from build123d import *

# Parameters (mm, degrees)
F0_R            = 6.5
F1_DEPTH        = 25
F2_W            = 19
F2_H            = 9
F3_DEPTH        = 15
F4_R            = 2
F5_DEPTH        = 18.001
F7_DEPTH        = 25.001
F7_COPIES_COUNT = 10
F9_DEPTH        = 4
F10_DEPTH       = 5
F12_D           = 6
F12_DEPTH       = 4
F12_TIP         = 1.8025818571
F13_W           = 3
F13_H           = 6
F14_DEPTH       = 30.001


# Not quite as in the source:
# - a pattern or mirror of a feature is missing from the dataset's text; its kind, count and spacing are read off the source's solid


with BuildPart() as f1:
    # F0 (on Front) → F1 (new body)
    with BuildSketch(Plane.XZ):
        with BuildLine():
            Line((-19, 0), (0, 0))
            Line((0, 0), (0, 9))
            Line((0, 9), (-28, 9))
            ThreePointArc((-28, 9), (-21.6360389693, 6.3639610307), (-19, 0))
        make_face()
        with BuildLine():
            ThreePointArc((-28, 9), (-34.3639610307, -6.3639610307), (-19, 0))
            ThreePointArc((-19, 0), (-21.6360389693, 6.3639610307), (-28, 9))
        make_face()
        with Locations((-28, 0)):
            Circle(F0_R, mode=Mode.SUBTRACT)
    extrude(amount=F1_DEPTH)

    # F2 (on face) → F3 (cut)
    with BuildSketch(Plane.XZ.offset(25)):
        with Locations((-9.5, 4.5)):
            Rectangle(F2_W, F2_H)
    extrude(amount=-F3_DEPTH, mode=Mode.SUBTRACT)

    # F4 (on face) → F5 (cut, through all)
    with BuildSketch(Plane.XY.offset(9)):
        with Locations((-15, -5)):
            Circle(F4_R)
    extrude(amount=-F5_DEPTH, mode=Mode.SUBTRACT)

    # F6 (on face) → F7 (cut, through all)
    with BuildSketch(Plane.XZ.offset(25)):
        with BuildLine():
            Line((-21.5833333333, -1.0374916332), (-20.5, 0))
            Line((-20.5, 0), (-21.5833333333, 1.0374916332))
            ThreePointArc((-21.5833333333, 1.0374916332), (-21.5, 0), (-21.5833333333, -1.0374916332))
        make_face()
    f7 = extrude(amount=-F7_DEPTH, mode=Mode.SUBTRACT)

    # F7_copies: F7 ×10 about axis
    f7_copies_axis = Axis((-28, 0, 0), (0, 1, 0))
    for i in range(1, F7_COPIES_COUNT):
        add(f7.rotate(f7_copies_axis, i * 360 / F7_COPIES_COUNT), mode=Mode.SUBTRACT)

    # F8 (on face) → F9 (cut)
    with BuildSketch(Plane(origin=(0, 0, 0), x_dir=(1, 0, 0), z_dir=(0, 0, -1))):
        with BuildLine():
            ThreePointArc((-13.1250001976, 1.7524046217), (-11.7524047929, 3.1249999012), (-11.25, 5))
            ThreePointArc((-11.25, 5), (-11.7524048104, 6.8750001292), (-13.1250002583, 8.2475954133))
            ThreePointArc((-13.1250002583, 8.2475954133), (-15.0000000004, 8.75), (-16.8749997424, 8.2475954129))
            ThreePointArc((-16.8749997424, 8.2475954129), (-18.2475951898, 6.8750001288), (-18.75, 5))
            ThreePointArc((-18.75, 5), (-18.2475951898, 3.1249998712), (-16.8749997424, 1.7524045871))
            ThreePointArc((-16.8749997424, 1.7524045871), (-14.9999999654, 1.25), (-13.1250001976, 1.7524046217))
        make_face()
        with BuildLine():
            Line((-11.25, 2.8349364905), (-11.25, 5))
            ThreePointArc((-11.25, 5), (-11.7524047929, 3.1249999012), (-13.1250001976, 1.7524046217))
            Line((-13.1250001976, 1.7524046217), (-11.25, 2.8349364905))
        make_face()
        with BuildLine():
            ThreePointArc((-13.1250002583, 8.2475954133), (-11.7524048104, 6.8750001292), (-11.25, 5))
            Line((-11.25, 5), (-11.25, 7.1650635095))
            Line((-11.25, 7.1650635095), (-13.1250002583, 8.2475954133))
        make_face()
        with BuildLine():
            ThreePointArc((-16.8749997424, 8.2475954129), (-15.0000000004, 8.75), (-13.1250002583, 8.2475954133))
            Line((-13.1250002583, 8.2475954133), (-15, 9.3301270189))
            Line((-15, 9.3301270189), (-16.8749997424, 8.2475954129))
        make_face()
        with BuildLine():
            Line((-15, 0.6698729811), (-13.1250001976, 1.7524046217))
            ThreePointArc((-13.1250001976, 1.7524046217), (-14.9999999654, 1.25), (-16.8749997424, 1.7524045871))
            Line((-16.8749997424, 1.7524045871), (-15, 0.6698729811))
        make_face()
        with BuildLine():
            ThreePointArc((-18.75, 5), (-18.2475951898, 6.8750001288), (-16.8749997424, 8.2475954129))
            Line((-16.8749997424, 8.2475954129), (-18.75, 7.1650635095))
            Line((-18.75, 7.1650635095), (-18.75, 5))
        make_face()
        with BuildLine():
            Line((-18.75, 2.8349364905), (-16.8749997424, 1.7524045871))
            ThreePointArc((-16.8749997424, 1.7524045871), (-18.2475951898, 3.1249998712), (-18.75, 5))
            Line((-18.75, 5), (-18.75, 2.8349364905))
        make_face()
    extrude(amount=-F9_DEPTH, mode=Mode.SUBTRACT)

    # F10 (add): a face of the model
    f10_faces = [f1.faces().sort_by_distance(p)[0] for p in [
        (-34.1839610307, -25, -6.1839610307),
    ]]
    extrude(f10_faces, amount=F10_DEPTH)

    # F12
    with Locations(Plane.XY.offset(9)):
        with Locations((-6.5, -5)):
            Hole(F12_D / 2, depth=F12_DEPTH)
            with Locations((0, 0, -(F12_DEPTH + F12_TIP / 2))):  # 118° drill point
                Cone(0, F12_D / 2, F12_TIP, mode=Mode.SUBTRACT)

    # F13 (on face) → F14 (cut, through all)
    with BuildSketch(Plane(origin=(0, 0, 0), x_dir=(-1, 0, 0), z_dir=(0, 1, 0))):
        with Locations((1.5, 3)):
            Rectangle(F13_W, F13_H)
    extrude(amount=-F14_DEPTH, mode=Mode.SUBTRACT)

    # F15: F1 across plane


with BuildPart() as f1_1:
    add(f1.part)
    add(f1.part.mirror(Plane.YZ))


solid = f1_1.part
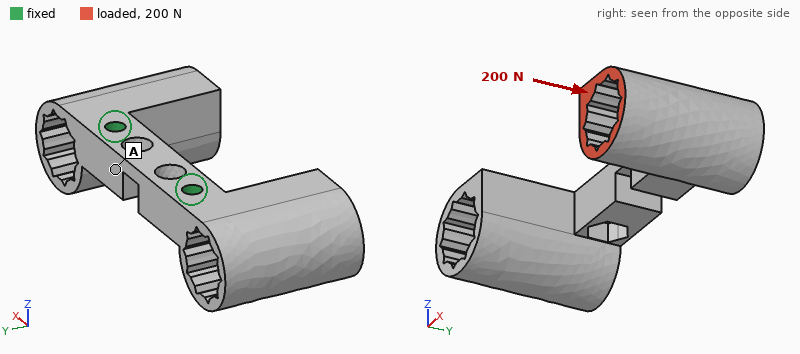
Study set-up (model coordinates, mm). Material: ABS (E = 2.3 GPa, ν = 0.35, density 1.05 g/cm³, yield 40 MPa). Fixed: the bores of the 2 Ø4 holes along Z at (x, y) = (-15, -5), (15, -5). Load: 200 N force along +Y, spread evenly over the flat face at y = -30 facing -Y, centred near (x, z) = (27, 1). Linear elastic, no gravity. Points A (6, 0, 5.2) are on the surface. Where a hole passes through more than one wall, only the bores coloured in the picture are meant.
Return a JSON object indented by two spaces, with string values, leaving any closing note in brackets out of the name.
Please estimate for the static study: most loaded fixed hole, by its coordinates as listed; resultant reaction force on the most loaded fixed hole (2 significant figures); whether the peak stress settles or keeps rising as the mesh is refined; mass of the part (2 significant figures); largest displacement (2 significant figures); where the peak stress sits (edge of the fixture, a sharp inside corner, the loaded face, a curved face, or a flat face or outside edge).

{
  "most loaded fixed hole, by its coordinates as listed": "(15, -5)",
  "resultant reaction force on the most loaded fixed hole": "220 N",
  "whether the peak stress settles or keeps rising as the mesh is refined": "keeps rising",
  "mass of the part": "11 g",
  "largest displacement": "0.85 mm",
  "where the peak stress sits": "edge of the fixture"
}
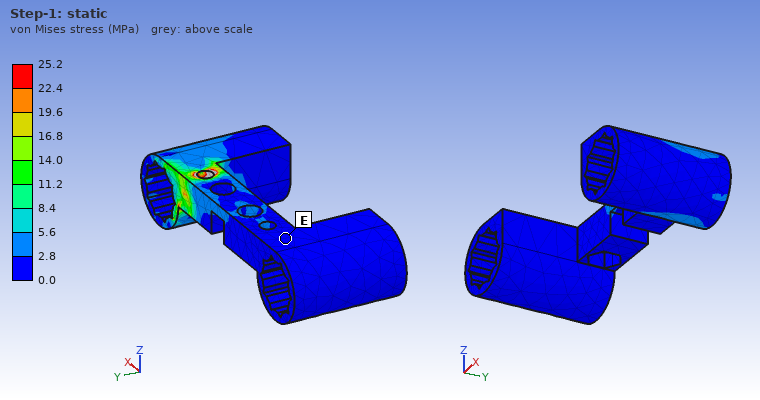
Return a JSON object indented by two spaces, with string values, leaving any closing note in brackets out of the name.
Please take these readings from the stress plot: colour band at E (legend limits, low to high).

{
  "colour band at E": "0.0 to 2.8 MPa"
}
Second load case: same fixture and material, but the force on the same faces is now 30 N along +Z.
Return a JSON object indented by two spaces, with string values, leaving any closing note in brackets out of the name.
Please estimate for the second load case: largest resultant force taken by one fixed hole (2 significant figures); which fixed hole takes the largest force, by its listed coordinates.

{
  "largest resultant force taken by one fixed hole": "32 N",
  "which fixed hole takes the largest force, by its listed coordinates": "(15, -5)"
}
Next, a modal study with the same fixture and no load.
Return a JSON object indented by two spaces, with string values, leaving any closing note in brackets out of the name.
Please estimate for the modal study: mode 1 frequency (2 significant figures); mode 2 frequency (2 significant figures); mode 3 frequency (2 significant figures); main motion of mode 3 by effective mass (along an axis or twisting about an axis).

{
  "mode 1 frequency": "1100 Hz",
  "mode 2 frequency": "1100 Hz",
  "mode 3 frequency": "1200 Hz",
  "main motion of mode 3 by effective mass": "along Y"
}
